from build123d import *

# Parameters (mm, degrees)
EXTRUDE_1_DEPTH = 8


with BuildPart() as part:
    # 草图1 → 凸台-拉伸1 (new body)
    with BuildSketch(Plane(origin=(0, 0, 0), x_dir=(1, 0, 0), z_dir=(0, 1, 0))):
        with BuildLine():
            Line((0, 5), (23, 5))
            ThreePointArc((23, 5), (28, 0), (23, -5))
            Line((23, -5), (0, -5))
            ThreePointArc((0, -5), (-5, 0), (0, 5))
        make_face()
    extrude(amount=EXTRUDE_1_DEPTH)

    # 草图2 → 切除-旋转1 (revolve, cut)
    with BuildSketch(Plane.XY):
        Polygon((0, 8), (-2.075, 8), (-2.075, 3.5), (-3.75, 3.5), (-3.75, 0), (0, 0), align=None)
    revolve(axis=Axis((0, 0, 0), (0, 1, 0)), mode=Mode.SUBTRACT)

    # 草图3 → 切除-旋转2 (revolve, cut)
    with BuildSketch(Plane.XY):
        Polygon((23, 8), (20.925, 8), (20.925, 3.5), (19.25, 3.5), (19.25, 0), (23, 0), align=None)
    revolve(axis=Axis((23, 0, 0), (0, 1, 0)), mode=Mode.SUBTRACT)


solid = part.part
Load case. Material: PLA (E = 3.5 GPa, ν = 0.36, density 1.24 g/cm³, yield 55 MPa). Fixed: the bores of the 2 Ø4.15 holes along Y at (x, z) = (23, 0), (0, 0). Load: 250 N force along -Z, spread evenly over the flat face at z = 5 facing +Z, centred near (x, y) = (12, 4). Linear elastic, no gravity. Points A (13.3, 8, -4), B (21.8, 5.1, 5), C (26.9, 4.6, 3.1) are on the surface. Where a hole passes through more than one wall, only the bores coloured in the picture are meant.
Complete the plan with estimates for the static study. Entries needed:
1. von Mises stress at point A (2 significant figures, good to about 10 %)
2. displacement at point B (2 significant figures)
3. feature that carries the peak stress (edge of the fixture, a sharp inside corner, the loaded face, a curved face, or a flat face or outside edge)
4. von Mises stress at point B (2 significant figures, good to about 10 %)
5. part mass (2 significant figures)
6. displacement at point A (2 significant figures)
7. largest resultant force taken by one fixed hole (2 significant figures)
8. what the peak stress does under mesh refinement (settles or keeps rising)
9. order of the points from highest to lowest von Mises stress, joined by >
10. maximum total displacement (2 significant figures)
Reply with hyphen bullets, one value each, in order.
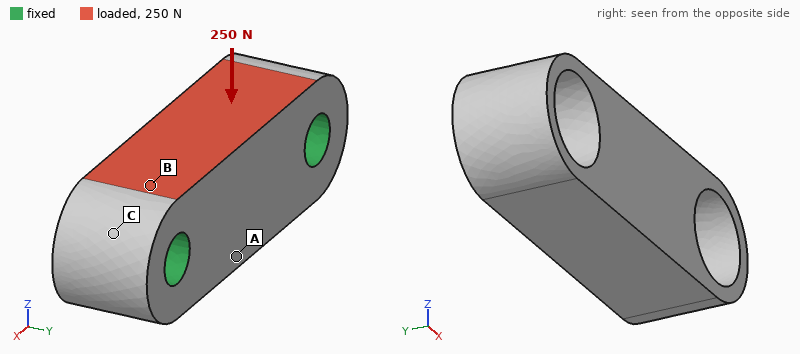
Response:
- 2.4 MPa
- 7.3 µm
- edge of the fixture
- 4.7 MPa
- 2.5 g
- 12 µm
- 130 N
- keeps rising
- B > A > C
- 28 µm
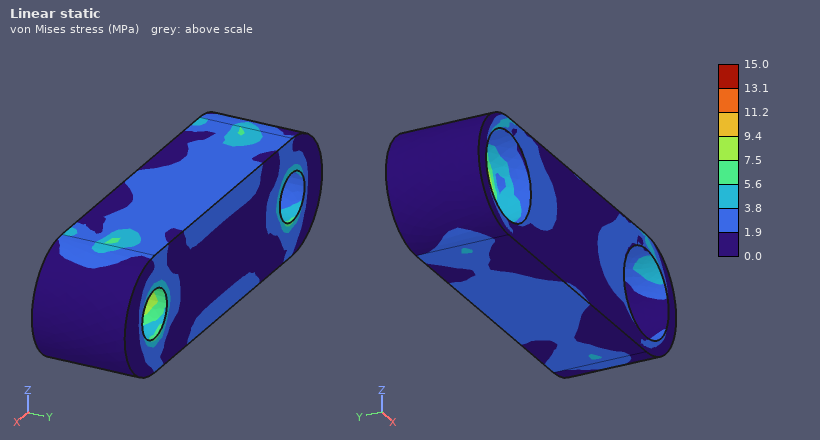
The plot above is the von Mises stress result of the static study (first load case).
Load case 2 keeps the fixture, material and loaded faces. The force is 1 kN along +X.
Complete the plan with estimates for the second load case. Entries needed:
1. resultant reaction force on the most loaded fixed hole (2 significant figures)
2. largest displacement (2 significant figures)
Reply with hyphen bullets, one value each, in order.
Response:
- 540 N
- 44 µm
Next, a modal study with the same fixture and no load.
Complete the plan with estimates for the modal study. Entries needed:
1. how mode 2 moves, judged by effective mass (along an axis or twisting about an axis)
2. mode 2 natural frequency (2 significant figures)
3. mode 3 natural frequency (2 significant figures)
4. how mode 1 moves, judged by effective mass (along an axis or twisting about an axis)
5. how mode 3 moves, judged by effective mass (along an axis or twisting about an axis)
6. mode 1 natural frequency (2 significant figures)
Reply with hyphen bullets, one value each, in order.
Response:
- along Y
- 15 kHz
- 18 kHz
- along Z
- along Z
- 12 kHz
